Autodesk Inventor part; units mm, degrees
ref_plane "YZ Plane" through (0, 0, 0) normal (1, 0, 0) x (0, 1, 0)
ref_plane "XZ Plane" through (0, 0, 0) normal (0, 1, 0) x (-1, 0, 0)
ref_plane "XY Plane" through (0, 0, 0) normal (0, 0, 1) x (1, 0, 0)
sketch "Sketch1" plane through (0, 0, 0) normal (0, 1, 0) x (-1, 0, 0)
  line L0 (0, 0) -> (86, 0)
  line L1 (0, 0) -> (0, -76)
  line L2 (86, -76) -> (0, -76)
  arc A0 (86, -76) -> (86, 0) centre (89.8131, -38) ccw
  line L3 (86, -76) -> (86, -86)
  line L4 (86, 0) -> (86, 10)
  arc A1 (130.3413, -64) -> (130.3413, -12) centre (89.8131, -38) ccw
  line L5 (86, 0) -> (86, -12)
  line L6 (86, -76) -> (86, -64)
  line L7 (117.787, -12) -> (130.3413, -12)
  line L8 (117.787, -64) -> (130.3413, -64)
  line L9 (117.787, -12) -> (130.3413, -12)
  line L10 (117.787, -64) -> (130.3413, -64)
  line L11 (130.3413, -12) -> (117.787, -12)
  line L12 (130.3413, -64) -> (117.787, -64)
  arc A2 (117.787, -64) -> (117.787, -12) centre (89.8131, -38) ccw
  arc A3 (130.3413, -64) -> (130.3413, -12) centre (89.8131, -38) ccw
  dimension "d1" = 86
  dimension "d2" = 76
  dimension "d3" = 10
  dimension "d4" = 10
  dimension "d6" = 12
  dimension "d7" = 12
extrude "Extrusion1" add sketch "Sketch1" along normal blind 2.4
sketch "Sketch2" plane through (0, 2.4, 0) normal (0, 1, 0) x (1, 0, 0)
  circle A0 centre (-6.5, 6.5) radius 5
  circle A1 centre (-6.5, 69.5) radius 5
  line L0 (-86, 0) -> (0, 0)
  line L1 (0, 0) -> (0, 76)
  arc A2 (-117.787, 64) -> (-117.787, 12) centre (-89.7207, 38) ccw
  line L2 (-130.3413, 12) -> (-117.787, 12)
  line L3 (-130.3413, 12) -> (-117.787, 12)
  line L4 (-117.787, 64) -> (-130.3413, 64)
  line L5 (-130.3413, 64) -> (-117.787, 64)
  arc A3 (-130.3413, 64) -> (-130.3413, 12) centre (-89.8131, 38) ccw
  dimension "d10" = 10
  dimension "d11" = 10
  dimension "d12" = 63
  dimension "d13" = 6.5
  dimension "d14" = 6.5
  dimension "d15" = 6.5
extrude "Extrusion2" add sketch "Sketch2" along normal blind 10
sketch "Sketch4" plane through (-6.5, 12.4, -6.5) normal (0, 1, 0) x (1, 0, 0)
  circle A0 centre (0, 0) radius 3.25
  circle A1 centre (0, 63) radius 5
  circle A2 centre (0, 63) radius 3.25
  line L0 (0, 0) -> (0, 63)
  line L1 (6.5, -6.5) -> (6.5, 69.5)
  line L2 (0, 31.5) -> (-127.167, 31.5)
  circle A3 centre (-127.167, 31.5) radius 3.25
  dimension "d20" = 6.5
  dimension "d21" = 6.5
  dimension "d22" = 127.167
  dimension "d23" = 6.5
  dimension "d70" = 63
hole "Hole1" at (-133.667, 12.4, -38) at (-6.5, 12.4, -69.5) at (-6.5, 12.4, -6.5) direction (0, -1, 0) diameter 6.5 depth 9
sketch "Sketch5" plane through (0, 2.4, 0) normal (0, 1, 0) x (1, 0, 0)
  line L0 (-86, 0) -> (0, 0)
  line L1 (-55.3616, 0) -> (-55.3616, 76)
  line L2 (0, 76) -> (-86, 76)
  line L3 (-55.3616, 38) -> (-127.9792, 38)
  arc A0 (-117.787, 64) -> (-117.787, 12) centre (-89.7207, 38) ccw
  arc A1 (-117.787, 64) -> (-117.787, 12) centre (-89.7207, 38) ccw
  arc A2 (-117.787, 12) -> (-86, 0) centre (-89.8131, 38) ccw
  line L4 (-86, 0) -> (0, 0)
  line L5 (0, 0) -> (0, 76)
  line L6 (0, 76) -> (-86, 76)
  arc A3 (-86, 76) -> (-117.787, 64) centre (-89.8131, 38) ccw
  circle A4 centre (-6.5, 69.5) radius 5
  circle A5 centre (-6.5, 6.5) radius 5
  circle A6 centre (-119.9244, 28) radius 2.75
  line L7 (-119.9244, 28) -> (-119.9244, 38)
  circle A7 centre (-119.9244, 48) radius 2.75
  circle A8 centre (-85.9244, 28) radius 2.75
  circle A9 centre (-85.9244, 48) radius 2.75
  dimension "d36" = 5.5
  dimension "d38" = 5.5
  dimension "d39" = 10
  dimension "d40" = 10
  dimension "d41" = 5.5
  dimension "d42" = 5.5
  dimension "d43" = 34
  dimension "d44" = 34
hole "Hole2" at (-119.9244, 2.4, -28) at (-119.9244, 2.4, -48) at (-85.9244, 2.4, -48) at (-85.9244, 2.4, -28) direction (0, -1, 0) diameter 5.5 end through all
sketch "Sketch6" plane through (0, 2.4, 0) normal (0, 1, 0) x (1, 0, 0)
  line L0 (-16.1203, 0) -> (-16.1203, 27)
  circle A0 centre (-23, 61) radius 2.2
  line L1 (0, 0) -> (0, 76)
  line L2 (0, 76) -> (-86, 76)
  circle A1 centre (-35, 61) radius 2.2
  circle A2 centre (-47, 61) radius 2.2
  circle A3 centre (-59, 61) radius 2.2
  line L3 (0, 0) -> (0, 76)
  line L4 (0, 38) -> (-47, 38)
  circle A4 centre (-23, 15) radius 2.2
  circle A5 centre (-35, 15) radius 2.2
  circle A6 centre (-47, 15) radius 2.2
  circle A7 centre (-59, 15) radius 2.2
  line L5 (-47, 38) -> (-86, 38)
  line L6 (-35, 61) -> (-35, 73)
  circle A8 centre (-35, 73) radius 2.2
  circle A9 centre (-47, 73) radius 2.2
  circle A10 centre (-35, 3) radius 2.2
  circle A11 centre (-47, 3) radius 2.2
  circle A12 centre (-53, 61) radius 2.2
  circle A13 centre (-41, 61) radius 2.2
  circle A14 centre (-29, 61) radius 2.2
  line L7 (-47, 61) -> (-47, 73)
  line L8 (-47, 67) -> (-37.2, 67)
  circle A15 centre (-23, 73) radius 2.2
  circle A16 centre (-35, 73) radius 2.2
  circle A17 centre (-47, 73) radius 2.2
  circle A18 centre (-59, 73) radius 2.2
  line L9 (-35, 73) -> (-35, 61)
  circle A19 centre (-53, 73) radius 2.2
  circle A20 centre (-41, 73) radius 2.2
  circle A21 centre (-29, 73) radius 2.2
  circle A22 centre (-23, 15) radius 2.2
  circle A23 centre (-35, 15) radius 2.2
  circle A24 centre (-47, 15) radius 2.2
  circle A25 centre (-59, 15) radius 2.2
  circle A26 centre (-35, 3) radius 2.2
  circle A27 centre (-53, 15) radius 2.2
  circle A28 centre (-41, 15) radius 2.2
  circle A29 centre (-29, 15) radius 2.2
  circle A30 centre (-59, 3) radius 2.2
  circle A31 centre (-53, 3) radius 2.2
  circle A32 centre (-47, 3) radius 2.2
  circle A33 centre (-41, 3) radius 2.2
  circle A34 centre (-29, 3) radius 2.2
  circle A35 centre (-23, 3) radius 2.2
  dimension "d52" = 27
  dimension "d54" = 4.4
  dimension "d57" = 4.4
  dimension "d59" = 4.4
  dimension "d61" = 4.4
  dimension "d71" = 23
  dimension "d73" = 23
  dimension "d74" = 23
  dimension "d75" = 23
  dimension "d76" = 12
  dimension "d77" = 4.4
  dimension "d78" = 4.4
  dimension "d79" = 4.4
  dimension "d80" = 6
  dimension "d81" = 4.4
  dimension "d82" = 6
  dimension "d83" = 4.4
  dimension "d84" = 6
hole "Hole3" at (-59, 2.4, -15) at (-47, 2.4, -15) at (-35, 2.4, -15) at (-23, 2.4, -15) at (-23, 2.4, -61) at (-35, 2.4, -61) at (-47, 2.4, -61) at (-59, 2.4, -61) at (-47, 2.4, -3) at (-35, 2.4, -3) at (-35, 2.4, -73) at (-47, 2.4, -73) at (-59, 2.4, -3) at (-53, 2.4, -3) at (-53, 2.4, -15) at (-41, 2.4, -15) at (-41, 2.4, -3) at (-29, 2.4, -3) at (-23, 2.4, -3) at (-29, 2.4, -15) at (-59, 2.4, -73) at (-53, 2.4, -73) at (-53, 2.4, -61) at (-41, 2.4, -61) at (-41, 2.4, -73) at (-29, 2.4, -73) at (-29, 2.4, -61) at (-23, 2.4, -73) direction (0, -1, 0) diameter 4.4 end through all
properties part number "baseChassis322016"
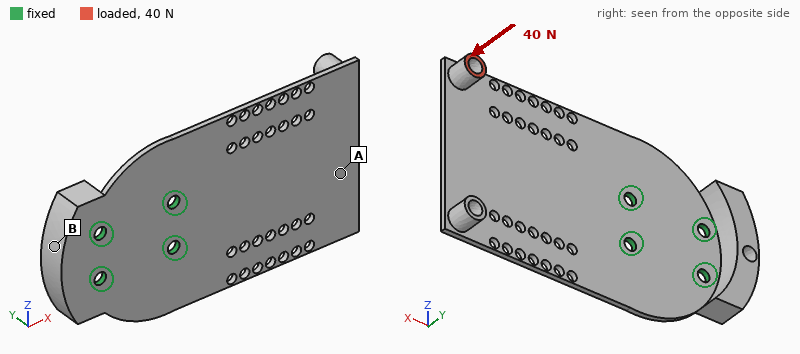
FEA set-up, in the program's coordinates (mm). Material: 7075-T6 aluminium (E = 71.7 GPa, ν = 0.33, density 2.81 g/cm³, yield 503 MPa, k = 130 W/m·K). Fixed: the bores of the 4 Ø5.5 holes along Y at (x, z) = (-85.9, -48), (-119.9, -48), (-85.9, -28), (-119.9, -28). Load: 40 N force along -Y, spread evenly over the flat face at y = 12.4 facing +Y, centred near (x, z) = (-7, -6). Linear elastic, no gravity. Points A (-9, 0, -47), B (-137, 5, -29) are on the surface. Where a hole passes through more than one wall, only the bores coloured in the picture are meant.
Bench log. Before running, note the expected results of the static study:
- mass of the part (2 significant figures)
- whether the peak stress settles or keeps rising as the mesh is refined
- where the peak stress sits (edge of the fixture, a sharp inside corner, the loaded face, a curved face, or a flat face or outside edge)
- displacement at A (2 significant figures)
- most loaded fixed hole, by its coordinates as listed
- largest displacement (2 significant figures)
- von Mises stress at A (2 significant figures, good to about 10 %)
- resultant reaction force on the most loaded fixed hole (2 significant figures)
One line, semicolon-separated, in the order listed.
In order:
79 g; keeps rising; edge of the fixture; 0.98 mm; (-85.9, -28); 1.7 mm; 13 MPa; 76 N
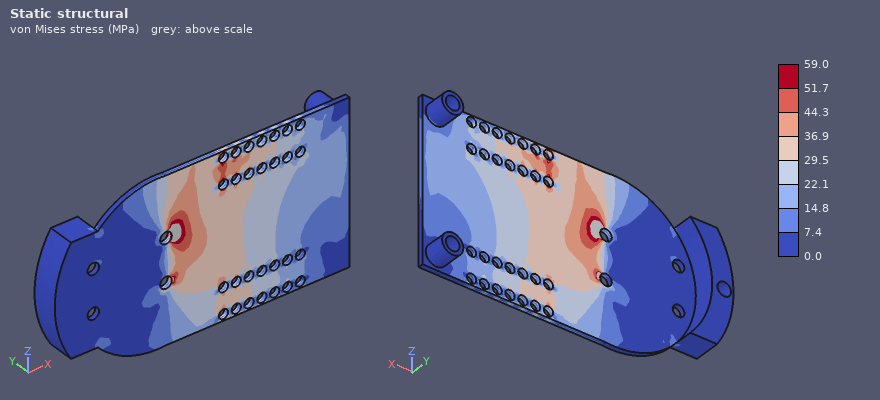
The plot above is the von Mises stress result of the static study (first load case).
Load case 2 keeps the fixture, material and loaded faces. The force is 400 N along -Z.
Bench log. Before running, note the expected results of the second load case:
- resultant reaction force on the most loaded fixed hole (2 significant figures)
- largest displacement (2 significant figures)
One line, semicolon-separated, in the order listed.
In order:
680 N; 1.7 mm
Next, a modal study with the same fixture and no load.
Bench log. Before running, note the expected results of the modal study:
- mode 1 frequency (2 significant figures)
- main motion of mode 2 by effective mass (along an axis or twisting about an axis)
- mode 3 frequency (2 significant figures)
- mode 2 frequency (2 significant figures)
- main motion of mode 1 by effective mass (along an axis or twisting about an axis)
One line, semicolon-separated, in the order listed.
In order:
240 Hz; twisting about X; 1500 Hz; 560 Hz; along Y
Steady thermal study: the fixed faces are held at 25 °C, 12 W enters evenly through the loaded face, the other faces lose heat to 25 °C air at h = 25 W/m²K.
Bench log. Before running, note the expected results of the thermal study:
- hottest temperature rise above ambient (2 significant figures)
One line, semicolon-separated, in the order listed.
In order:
71 K
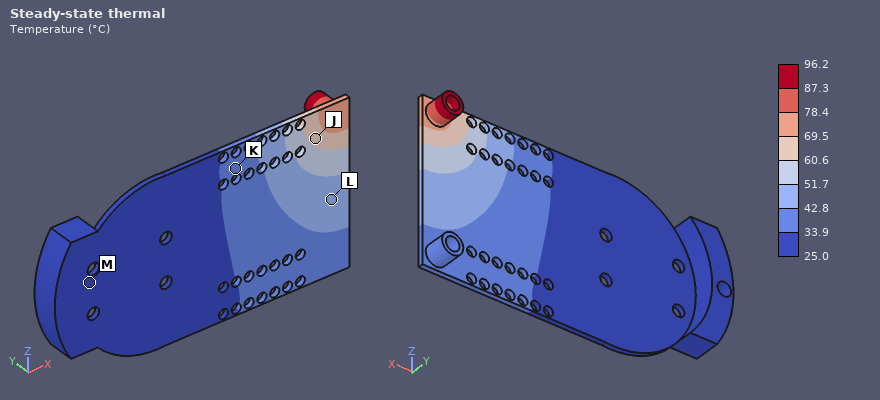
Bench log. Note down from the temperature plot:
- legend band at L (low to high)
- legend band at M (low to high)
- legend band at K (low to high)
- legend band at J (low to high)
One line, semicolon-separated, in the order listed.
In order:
42.8 to 51.7 °C; 25.0 to 33.9 °C; 33.9 to 42.8 °C; 60.6 to 69.5 °C
